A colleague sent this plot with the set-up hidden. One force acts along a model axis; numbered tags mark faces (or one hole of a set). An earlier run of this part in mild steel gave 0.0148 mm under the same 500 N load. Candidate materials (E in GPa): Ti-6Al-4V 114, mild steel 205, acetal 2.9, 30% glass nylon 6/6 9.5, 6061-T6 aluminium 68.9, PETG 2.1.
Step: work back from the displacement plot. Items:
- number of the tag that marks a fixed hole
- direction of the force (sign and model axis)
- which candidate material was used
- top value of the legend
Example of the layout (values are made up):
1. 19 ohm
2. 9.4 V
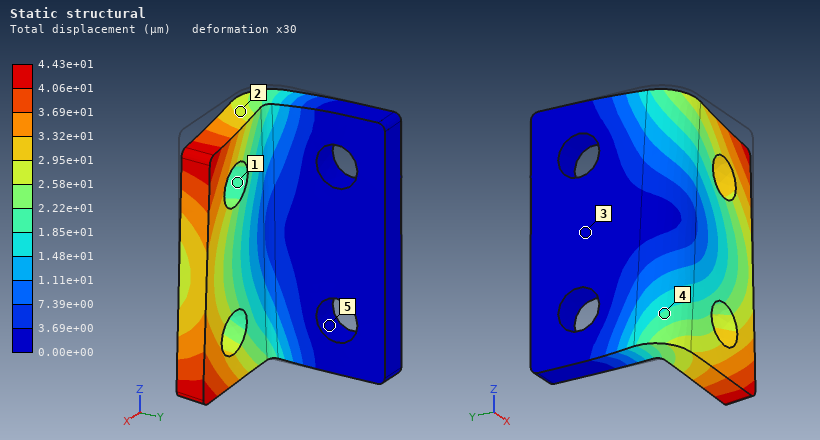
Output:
1. 5
2. -Z
3. 6061-T6 aluminium
4. 4.43e+01 µm
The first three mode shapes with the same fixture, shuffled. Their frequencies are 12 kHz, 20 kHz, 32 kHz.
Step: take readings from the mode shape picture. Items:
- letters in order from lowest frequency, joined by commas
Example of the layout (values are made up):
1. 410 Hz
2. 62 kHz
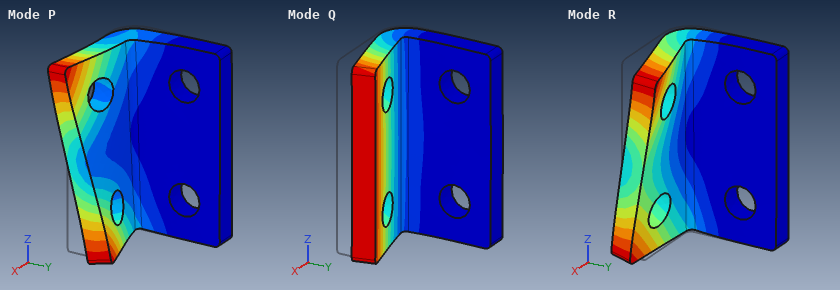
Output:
1. Q, R, P
